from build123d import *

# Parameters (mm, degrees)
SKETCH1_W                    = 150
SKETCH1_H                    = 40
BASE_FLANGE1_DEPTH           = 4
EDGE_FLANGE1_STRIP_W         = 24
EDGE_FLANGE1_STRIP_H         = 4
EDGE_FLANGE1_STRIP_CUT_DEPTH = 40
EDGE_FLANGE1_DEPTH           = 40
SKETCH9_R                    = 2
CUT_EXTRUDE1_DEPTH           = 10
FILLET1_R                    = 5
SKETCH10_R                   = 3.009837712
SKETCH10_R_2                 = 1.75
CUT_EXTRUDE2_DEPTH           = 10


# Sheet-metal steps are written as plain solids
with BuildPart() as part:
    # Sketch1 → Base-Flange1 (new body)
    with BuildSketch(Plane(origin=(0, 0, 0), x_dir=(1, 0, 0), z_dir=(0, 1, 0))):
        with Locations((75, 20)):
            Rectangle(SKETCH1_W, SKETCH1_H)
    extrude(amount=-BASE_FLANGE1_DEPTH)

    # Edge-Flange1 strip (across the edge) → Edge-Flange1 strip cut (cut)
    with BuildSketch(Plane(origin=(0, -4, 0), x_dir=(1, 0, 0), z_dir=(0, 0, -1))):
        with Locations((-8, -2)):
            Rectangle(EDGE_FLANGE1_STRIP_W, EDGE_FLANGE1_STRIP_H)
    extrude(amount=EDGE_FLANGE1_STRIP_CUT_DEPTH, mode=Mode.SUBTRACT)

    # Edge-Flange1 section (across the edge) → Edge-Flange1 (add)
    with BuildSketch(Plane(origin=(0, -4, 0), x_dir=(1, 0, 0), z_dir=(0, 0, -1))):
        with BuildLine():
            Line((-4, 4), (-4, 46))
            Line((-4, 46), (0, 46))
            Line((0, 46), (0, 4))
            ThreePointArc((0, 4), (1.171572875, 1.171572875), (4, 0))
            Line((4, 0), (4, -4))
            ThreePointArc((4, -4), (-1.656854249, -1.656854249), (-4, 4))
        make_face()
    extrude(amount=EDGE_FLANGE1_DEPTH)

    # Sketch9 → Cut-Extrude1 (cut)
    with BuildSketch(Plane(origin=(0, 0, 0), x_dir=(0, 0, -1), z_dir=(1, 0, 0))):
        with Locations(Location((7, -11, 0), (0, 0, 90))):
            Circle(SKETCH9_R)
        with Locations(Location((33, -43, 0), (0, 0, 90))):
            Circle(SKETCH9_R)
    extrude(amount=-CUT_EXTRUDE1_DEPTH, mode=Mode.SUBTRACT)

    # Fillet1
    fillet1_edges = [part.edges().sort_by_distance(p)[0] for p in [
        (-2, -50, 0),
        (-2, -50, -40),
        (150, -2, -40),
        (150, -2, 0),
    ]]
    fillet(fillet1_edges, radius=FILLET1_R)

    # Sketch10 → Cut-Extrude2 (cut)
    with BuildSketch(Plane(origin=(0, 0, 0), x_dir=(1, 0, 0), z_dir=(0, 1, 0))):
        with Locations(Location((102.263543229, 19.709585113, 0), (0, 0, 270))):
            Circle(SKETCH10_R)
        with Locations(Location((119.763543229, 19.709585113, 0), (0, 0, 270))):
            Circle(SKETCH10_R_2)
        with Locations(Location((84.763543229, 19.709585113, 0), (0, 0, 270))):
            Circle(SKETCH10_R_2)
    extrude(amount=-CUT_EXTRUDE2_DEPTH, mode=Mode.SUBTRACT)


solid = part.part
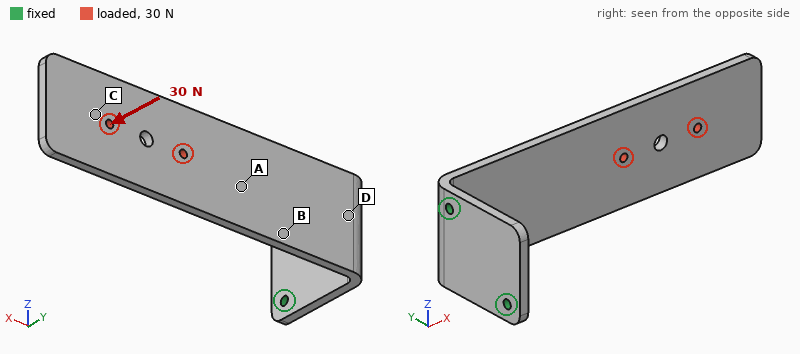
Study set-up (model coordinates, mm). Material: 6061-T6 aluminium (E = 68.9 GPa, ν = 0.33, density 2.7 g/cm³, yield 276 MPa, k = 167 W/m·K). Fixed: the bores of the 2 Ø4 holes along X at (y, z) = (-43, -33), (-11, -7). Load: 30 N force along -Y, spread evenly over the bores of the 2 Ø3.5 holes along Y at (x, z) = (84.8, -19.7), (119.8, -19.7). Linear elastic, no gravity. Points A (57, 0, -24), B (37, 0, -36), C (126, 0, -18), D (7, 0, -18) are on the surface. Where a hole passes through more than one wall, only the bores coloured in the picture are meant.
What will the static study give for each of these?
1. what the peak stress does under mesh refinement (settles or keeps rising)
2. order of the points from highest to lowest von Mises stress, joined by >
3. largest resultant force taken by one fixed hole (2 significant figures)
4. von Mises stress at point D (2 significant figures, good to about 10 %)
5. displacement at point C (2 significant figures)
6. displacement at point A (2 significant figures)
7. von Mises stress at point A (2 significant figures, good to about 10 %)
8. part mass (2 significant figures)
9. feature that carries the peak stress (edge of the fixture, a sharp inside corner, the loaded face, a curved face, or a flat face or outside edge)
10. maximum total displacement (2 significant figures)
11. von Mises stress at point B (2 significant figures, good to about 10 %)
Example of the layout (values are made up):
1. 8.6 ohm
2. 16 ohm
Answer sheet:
1. keeps rising
2. D > B > A > C
3. 46 N
4. 25 MPa
5. 1.3 mm
6. 0.42 mm
7. 13 MPa
8. 84 g
9. edge of the fixture
10. 1.6 mm
11. 18 MPa
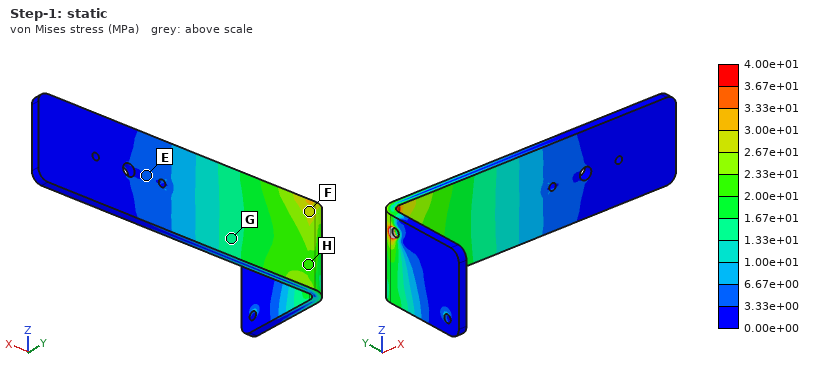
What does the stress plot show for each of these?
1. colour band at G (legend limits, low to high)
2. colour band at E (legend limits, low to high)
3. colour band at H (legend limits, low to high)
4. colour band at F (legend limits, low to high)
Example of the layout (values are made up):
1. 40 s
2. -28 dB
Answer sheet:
1. 1.33e+01 to 1.67e+01 MPa
2. 3.33e+00 to 6.67e+00 MPa
3. 2.00e+01 to 2.33e+01 MPa
4. 2.67e+01 to 3.00e+01 MPa
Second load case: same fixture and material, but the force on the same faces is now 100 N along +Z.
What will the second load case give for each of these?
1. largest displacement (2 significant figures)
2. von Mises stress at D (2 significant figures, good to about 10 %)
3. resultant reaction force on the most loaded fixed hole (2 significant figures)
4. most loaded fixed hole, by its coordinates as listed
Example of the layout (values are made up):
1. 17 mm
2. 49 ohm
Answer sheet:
1. 0.92 mm
2. 21 MPa
3. 120 N
4. (-11, -7)
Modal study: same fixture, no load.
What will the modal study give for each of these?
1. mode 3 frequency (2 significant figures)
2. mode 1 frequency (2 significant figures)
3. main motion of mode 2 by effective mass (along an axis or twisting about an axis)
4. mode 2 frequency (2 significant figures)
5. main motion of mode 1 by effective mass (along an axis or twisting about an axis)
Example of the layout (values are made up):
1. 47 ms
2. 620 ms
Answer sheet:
1. 820 Hz
2. 130 Hz
3. along Z
4. 310 Hz
5. along Y
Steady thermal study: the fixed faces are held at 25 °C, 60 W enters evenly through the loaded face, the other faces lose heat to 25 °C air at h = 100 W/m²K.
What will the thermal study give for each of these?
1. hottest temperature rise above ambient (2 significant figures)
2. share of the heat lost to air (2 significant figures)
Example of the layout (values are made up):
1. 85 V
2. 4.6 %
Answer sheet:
1. 71 K
2. 86 %
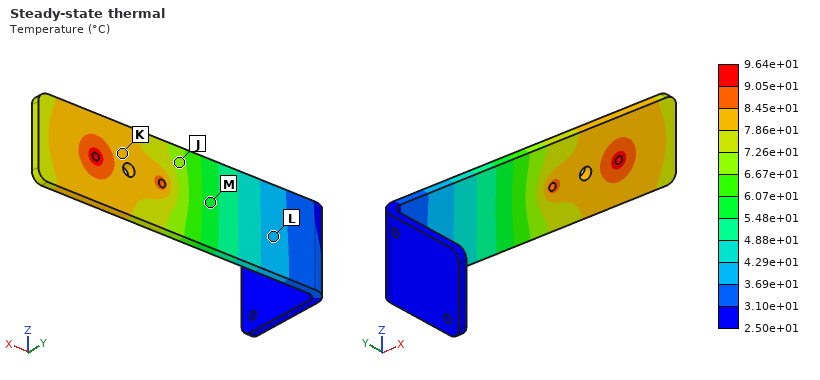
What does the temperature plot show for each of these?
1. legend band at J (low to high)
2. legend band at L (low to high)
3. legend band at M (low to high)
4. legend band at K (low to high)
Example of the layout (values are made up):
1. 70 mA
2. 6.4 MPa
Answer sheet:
1. 6.67e+01 to 7.26e+01 °C
2. 3.69e+01 to 4.29e+01 °C
3. 5.48e+01 to 6.07e+01 °C
4. 7.86e+01 to 8.45e+01 °C
